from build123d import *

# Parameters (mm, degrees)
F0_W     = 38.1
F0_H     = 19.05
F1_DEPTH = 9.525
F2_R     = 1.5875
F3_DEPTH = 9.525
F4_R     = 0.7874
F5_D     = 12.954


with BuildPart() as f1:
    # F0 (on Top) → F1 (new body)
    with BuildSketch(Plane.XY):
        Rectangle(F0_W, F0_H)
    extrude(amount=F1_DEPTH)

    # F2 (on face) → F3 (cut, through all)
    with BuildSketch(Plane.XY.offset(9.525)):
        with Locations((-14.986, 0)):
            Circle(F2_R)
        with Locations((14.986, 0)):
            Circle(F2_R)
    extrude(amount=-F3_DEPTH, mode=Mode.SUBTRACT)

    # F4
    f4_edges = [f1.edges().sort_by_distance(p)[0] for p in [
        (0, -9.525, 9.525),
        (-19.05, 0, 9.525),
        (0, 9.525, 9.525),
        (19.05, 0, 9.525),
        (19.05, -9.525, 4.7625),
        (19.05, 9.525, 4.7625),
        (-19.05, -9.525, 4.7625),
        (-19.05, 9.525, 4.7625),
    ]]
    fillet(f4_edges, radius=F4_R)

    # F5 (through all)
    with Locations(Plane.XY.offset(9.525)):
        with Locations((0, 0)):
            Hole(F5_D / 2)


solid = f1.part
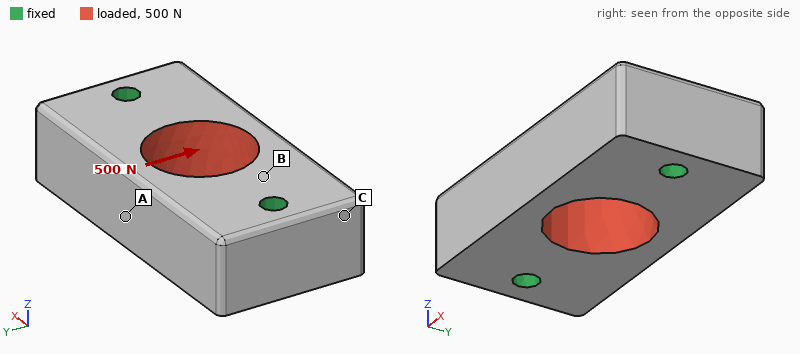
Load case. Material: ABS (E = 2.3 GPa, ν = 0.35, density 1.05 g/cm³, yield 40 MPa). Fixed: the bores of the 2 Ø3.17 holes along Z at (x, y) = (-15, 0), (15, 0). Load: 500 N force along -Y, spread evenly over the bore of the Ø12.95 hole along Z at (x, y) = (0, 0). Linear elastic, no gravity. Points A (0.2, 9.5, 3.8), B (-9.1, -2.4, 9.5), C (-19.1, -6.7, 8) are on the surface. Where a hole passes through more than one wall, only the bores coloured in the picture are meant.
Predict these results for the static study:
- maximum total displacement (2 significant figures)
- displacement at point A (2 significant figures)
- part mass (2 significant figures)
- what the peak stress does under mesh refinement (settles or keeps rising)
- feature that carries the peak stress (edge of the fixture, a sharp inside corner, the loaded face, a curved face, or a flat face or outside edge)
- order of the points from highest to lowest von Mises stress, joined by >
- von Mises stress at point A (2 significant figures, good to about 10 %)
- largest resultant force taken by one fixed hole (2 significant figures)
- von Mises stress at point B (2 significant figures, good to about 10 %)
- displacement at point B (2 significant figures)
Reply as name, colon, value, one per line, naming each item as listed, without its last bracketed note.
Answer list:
maximum total displacement: 47 µm
displacement at point A: 42 µm
part mass: 5.8 g
what the peak stress does under mesh refinement: keeps rising
feature that carries the peak stress: edge of the fixture
order of the points from highest to lowest von Mises stress, joined by >: A > B > C
von Mises stress at point A: 7.3 MPa
largest resultant force taken by one fixed hole: 250 N
von Mises stress at point B: 3.6 MPa
displacement at point B: 20 µm
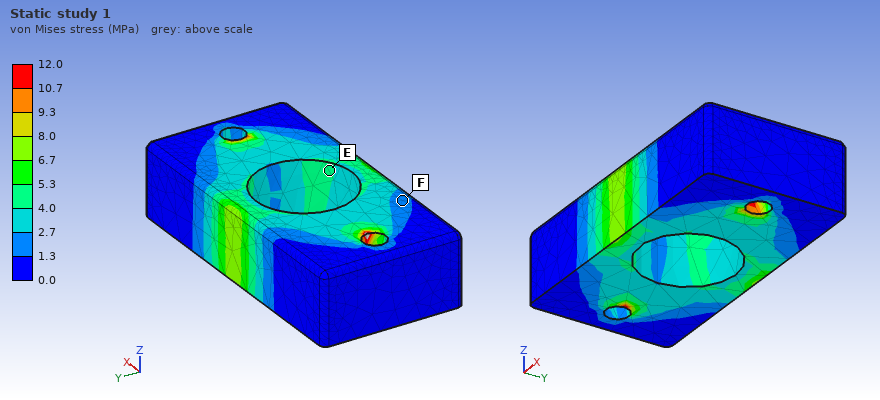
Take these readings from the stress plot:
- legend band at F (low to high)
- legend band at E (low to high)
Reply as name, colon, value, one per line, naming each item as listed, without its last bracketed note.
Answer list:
legend band at F: 1.3 to 2.7 MPa
legend band at E: 4.0 to 5.3 MPa
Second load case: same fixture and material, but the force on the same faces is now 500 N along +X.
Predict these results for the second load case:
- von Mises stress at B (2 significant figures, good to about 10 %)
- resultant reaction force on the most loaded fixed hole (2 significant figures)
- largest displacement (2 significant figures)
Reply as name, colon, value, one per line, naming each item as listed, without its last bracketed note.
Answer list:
von Mises stress at B: 2.5 MPa
resultant reaction force on the most loaded fixed hole: 250 N
largest displacement: 16 µm
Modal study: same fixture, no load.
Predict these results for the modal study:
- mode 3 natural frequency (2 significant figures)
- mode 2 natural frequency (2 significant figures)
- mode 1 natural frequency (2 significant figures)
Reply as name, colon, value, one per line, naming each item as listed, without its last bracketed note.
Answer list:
mode 3 natural frequency: 10 kHz
mode 2 natural frequency: 9800 Hz
mode 1 natural frequency: 9700 Hz
